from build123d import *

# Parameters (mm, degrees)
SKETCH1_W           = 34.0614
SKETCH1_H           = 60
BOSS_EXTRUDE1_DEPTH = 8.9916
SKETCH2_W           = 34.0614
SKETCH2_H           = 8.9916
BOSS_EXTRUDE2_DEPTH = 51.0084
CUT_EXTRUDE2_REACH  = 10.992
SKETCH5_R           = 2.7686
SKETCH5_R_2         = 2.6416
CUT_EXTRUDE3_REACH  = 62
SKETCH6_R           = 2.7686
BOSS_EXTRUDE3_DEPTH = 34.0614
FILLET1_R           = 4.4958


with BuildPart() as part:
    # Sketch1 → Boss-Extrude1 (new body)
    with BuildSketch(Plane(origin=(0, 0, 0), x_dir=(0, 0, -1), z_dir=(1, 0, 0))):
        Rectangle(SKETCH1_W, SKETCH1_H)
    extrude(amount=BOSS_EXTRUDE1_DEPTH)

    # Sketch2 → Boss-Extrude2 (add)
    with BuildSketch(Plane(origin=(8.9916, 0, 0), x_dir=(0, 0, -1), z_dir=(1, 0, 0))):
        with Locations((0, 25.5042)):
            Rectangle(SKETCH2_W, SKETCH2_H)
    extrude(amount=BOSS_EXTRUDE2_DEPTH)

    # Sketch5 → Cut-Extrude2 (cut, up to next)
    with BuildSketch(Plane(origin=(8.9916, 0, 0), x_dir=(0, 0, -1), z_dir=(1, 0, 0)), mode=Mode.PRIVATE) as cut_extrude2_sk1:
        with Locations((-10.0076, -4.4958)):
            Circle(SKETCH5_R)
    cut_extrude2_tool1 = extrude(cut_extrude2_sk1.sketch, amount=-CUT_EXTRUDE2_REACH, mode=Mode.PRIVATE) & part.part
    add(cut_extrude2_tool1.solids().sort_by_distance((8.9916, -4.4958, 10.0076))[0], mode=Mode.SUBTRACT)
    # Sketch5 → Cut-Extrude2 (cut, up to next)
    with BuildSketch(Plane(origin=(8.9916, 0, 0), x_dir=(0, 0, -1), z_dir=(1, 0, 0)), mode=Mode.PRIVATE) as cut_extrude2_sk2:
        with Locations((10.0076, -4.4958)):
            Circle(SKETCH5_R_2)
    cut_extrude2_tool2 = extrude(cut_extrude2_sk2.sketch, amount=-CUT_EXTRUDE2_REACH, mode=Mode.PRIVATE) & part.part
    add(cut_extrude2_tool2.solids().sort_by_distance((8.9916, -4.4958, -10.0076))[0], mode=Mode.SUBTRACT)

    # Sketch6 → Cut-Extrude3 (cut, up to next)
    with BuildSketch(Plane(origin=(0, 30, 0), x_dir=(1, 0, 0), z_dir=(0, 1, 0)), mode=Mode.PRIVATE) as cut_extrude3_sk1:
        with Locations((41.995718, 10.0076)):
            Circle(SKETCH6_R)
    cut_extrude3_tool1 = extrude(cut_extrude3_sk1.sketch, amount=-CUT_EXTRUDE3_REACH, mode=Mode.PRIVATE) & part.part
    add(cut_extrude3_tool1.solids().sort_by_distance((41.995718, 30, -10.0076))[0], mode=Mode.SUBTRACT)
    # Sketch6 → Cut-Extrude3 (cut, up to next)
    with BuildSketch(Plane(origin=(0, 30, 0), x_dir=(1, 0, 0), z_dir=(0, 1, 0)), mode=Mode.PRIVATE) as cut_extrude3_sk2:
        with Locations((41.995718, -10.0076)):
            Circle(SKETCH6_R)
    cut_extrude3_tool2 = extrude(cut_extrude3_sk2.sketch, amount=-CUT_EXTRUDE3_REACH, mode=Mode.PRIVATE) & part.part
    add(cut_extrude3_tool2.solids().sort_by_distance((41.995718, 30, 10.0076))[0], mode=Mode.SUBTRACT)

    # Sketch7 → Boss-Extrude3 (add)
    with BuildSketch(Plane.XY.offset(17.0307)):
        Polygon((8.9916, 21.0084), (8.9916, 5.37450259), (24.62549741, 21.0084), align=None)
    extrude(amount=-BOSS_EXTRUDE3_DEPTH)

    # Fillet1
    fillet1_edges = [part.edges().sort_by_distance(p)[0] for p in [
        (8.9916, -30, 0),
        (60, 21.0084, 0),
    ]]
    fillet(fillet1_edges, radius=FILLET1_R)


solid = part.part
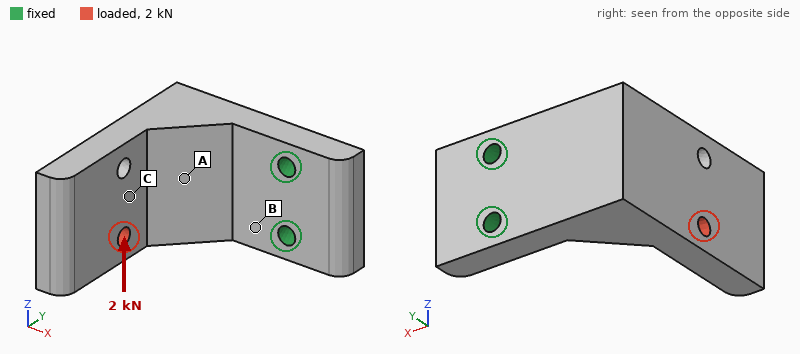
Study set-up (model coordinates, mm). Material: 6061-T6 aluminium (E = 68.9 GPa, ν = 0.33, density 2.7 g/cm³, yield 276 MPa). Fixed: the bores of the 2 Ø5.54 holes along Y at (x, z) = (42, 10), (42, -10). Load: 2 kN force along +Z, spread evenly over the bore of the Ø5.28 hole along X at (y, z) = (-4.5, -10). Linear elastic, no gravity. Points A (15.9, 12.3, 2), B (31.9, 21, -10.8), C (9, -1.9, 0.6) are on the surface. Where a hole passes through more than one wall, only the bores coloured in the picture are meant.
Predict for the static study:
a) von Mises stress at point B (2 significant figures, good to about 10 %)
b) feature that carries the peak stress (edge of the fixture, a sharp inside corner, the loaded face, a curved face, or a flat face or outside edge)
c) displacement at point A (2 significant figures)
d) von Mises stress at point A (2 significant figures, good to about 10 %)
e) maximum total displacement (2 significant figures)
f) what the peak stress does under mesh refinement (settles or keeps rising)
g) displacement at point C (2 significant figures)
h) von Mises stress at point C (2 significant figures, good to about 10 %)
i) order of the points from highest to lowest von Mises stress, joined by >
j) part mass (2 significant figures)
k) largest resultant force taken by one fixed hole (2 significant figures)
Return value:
73 MPa
edge of the fixture
0.066 mm
37 MPa
0.26 mm
keeps rising
0.13 mm
17 MPa
B > A > C
100 g
4.1 kN
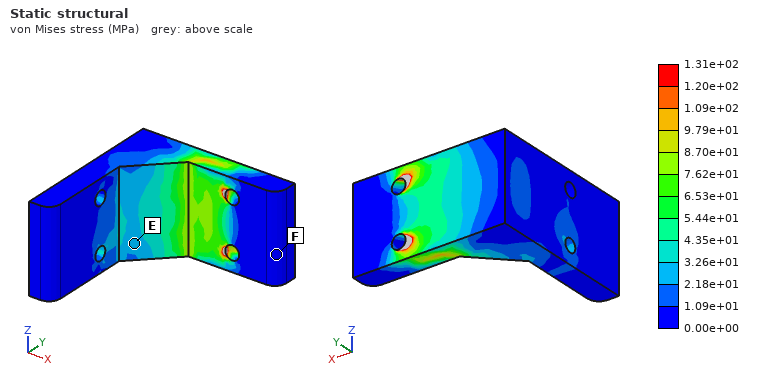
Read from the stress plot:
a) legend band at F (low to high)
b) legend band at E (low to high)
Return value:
0.00e+00 to 1.09e+01 MPa
2.18e+01 to 3.26e+01 MPa
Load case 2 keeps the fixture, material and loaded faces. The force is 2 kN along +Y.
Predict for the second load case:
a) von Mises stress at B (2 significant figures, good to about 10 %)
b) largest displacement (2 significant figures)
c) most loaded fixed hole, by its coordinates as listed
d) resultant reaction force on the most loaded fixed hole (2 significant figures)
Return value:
130 MPa
0.54 mm
(42, -10)
1.8 kN
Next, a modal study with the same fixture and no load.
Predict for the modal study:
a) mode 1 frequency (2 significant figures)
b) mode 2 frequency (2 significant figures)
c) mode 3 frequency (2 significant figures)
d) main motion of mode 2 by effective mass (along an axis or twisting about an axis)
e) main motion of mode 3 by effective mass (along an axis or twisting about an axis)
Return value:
1400 Hz
2500 Hz
4900 Hz
along Z
along Y
